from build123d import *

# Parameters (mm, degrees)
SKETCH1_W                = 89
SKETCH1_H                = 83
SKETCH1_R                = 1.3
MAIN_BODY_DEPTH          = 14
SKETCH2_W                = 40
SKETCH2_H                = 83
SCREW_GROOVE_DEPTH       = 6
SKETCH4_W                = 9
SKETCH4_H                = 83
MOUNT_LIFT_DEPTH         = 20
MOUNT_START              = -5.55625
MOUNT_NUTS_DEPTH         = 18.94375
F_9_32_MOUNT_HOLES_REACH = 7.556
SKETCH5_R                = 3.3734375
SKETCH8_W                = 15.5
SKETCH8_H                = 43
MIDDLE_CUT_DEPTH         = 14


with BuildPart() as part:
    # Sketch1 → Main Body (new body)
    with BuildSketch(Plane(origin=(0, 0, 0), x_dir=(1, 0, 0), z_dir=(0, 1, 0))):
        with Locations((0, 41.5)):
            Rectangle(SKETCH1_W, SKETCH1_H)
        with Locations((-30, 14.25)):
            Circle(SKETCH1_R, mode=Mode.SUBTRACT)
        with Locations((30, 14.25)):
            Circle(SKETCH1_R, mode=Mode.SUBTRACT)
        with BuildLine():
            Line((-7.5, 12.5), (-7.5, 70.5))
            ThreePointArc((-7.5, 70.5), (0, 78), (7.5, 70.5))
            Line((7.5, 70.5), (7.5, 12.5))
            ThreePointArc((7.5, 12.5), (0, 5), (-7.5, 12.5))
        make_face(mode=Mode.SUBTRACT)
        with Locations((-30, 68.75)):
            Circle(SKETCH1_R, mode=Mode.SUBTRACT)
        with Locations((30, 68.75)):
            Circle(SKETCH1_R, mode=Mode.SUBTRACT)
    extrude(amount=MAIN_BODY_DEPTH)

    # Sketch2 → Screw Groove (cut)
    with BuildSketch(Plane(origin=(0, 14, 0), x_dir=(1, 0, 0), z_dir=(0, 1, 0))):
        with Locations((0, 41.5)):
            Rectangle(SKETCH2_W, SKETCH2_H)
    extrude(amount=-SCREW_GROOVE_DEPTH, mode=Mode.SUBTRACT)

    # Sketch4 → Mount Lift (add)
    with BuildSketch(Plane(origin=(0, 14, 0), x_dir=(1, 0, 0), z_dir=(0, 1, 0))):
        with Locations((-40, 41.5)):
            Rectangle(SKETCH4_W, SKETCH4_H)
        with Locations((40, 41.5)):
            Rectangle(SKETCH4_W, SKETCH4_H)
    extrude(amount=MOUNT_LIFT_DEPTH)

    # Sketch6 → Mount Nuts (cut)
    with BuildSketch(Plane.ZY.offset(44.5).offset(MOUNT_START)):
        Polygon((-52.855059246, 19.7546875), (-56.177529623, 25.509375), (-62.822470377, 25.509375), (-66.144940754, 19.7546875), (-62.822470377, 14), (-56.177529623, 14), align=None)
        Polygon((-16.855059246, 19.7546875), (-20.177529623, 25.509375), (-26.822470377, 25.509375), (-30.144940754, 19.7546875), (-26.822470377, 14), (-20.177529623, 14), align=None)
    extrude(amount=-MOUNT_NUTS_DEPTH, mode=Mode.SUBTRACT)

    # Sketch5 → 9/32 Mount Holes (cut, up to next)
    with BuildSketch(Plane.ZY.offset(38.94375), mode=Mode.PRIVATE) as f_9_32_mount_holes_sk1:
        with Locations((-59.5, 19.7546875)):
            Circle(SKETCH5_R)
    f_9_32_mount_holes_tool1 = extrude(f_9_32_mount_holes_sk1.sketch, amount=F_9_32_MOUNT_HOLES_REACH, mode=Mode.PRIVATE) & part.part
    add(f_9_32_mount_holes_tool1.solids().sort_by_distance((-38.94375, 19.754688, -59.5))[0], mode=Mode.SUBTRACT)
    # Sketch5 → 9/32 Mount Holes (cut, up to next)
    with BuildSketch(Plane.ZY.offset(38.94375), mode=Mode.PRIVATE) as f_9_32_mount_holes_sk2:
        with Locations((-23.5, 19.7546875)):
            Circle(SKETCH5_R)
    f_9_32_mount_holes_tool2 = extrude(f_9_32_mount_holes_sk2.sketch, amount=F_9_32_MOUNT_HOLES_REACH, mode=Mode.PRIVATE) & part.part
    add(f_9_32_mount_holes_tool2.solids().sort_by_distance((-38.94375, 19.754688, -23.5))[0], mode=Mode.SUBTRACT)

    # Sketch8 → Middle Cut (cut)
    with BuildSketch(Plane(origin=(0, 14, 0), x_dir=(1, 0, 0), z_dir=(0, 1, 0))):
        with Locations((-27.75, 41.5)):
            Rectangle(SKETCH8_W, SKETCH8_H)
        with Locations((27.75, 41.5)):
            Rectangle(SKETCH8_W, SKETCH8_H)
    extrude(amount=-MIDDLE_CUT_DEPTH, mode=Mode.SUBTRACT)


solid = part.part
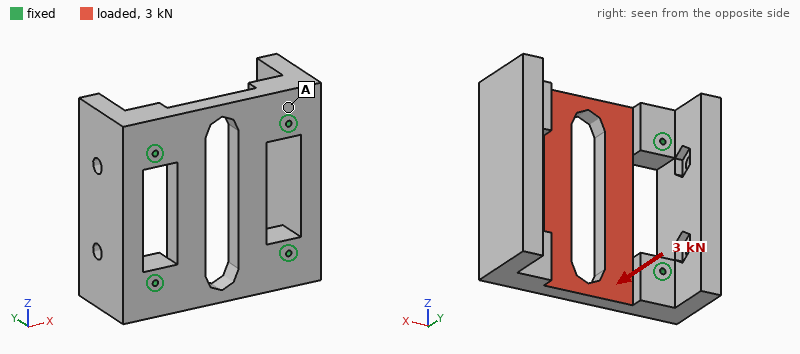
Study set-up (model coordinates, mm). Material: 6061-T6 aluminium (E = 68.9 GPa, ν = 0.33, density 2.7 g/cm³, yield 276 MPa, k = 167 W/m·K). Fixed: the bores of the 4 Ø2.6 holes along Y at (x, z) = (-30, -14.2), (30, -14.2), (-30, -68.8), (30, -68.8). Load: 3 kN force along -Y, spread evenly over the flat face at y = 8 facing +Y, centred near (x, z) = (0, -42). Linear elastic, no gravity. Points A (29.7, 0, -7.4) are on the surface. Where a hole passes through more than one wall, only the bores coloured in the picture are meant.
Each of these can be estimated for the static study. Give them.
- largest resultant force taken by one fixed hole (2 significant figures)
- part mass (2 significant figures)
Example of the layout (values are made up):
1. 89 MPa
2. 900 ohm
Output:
1. 760 N
2. 230 g
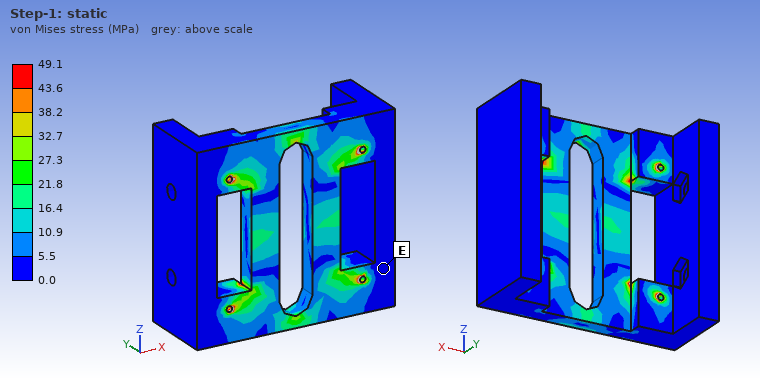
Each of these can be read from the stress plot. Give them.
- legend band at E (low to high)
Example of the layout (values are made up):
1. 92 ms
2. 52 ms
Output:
1. 0.0 to 5.5 MPa
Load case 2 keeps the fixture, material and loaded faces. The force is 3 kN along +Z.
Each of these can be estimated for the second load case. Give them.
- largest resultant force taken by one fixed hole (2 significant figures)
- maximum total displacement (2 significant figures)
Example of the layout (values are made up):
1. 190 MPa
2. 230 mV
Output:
1. 800 N
2. 8.7 µm
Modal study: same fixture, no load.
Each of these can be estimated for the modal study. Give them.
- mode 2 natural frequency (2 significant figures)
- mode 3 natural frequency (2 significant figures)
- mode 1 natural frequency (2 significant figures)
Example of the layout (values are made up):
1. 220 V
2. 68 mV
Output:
1. 6200 Hz
2. 8800 Hz
3. 6000 Hz
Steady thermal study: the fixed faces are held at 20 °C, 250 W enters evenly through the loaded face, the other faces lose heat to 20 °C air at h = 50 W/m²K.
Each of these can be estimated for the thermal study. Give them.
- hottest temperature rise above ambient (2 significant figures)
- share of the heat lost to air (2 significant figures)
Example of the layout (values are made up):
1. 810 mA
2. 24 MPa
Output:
1. 55 K
2. 5.7 %
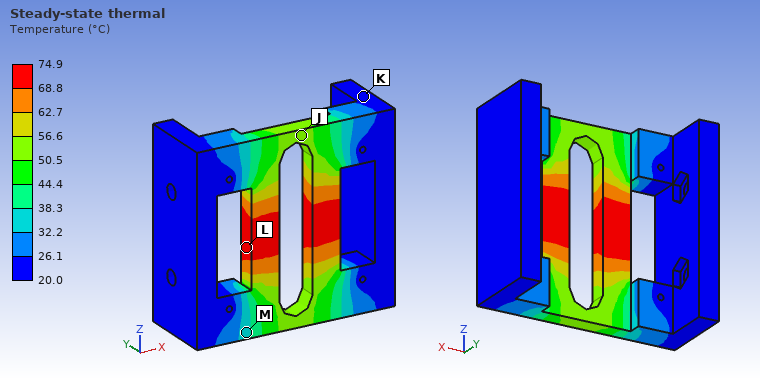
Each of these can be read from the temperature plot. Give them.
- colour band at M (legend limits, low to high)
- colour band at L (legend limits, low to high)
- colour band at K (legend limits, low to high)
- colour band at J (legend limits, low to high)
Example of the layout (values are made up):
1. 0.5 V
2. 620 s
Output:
1. 32.2 to 38.3 °C
2. 68.8 to 74.9 °C
3. 20.0 to 26.1 °C
4. 50.5 to 56.6 °C
